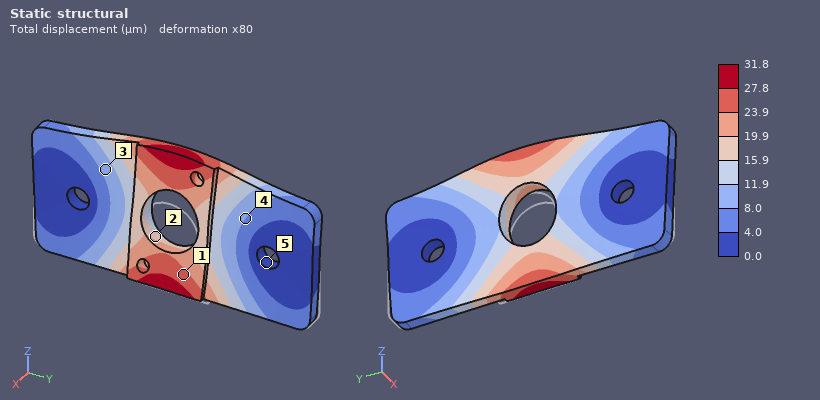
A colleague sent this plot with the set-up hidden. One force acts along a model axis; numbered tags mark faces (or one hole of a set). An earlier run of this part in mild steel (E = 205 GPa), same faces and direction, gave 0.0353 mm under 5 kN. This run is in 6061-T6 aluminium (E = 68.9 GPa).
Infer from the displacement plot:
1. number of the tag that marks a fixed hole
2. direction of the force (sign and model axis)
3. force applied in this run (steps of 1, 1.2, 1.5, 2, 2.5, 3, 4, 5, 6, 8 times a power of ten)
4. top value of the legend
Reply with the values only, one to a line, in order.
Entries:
5
+Z
1.5 kN
31.8 µm
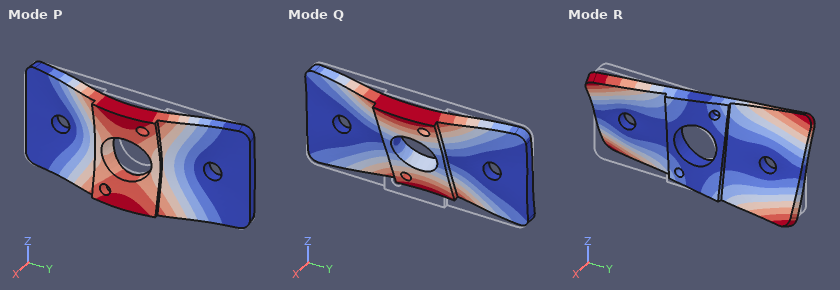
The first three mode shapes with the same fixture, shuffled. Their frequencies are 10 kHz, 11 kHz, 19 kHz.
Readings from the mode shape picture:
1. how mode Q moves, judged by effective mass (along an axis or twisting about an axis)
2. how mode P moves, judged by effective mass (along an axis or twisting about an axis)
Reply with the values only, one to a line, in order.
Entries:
twisting about Y
along X
